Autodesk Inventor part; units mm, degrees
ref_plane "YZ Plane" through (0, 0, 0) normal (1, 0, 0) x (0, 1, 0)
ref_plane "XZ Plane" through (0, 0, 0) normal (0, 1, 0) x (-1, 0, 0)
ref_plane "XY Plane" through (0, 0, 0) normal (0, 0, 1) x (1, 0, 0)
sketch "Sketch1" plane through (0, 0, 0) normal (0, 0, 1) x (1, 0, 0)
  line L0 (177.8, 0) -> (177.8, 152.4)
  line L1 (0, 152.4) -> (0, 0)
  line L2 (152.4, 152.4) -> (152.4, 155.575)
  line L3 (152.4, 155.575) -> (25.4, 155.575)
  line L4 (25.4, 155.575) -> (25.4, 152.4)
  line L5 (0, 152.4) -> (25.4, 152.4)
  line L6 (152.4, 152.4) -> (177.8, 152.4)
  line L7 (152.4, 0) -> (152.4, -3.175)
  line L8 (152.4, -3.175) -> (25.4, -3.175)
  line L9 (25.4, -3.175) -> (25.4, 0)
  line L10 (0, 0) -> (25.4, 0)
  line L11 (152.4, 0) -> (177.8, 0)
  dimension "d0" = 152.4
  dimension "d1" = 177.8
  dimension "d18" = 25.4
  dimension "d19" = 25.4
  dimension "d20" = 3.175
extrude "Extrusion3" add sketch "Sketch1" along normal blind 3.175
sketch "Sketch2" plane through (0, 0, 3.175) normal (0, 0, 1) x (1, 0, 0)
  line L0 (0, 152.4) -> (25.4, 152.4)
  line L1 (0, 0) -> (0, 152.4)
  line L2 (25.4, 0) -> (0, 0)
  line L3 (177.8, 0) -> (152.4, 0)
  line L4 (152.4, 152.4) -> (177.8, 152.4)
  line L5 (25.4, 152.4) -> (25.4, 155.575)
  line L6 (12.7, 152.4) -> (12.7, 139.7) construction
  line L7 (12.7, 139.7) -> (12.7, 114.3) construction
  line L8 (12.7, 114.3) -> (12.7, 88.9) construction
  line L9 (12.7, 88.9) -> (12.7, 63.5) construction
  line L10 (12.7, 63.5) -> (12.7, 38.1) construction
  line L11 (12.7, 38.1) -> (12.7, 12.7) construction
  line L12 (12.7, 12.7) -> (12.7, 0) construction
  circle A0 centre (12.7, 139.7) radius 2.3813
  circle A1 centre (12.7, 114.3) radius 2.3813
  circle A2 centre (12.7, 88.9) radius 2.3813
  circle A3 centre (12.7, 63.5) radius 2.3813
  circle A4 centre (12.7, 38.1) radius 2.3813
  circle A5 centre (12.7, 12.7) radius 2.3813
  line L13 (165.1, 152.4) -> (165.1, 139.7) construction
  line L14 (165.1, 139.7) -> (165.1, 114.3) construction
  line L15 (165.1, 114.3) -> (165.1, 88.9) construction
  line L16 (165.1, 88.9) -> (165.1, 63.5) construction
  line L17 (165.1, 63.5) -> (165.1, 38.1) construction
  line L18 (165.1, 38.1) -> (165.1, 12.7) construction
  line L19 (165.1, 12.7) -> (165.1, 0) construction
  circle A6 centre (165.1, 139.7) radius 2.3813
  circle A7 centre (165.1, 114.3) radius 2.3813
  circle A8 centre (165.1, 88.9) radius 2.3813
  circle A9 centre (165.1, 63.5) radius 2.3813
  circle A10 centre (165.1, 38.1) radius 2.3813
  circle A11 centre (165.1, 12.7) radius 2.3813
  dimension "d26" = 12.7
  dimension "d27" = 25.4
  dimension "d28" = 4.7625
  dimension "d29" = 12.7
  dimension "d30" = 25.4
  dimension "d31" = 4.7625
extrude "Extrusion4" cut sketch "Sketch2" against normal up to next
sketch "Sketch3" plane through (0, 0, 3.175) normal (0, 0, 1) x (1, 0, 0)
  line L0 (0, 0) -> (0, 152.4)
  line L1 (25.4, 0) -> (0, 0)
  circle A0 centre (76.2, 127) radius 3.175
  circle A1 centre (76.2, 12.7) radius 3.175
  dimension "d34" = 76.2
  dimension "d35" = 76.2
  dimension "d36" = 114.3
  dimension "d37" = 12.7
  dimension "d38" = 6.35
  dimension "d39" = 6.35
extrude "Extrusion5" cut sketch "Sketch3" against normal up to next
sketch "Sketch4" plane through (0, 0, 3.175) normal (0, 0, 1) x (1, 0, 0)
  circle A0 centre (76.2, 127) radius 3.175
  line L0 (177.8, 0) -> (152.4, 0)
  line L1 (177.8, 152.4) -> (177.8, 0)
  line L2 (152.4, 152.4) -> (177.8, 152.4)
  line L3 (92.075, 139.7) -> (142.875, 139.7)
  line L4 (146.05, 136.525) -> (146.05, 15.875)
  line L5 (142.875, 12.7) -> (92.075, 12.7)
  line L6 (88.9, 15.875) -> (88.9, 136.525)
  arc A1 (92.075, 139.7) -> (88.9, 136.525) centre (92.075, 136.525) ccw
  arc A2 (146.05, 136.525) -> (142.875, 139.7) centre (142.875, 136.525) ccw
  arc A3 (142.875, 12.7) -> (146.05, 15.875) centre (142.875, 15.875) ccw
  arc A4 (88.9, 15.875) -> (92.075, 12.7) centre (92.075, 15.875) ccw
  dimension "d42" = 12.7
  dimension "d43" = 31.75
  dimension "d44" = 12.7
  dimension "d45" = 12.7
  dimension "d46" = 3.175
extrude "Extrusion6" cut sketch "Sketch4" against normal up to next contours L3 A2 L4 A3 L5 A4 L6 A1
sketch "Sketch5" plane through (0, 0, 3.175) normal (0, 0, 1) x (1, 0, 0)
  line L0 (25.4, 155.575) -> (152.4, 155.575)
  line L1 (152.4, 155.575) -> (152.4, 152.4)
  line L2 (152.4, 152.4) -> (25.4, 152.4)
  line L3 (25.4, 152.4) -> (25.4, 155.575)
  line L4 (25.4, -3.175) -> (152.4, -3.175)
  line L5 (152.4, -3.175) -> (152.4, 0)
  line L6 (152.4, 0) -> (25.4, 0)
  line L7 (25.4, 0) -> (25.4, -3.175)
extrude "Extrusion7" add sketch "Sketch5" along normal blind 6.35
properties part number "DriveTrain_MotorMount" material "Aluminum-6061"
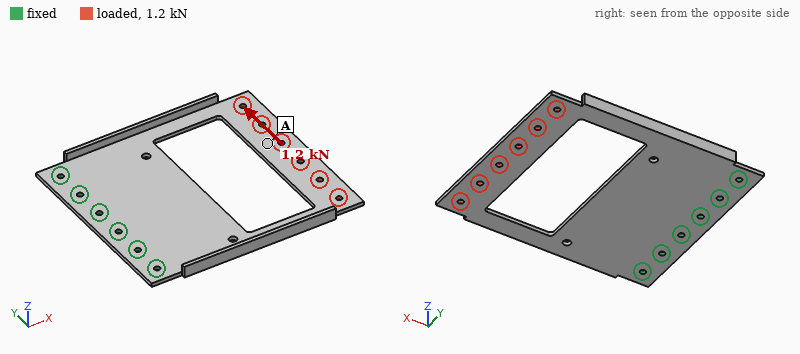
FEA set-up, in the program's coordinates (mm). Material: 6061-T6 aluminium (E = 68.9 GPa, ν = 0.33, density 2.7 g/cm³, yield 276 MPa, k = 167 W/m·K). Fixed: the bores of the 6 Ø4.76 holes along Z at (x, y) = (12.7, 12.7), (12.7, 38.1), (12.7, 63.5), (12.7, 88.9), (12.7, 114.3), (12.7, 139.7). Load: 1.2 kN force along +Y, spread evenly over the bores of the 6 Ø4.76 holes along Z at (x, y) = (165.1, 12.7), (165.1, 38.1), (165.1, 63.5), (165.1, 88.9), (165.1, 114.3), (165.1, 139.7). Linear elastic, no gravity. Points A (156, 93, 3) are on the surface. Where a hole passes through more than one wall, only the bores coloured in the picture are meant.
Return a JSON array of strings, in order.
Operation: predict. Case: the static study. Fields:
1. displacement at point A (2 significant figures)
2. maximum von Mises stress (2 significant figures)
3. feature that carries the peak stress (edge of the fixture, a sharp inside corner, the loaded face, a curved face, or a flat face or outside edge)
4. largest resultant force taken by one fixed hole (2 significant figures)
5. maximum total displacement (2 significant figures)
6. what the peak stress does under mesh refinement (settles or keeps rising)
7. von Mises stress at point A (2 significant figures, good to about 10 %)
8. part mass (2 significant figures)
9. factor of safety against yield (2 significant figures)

["0.38 mm", "270 MPa", "a curved face", "1.2 kN", "0.49 mm", "settles", "15 MPa", "190 g", "1.0"]
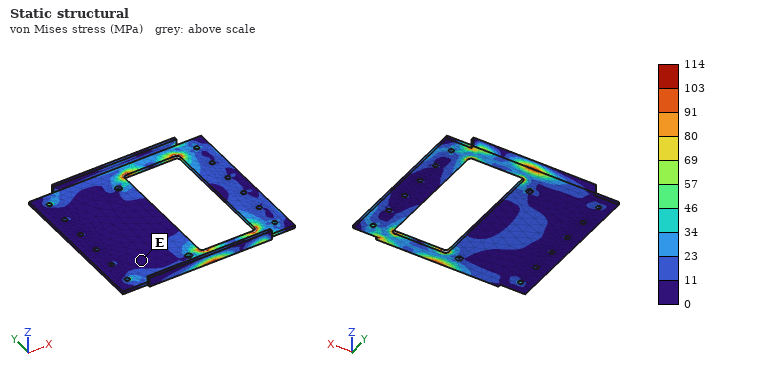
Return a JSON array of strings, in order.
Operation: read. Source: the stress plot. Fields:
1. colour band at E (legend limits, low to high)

["0 to 11 MPa"]
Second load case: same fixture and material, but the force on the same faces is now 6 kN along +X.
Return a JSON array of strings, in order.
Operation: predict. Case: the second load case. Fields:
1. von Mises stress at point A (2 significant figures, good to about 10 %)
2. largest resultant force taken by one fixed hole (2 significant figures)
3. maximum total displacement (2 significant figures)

["41 MPa", "2.1 kN", "0.89 mm"]
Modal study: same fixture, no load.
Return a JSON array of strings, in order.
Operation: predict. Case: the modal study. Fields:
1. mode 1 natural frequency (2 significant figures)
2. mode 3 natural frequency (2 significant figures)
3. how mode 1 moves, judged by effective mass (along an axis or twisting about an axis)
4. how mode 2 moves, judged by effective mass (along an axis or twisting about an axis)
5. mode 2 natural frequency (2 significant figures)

["130 Hz", "590 Hz", "along Z", "twisting about X", "230 Hz"]
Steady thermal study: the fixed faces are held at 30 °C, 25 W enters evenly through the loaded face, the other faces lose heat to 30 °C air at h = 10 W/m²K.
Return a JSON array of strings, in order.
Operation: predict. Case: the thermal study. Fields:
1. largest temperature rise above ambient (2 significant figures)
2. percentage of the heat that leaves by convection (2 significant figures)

["85 K", "49 %"]
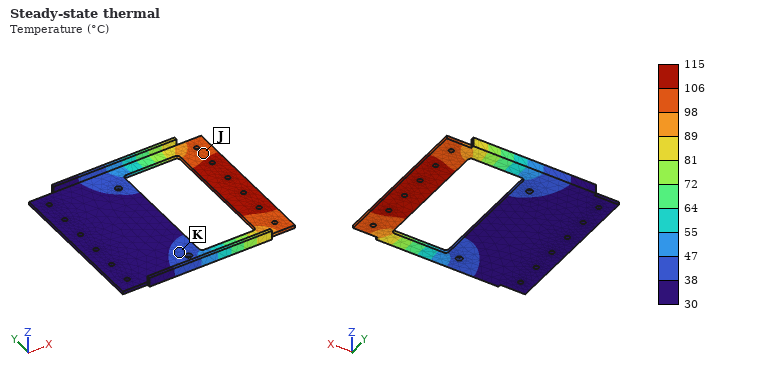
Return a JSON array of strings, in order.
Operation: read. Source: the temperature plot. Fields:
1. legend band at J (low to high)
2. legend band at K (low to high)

["98 to 106 °C", "38 to 47 °C"]
